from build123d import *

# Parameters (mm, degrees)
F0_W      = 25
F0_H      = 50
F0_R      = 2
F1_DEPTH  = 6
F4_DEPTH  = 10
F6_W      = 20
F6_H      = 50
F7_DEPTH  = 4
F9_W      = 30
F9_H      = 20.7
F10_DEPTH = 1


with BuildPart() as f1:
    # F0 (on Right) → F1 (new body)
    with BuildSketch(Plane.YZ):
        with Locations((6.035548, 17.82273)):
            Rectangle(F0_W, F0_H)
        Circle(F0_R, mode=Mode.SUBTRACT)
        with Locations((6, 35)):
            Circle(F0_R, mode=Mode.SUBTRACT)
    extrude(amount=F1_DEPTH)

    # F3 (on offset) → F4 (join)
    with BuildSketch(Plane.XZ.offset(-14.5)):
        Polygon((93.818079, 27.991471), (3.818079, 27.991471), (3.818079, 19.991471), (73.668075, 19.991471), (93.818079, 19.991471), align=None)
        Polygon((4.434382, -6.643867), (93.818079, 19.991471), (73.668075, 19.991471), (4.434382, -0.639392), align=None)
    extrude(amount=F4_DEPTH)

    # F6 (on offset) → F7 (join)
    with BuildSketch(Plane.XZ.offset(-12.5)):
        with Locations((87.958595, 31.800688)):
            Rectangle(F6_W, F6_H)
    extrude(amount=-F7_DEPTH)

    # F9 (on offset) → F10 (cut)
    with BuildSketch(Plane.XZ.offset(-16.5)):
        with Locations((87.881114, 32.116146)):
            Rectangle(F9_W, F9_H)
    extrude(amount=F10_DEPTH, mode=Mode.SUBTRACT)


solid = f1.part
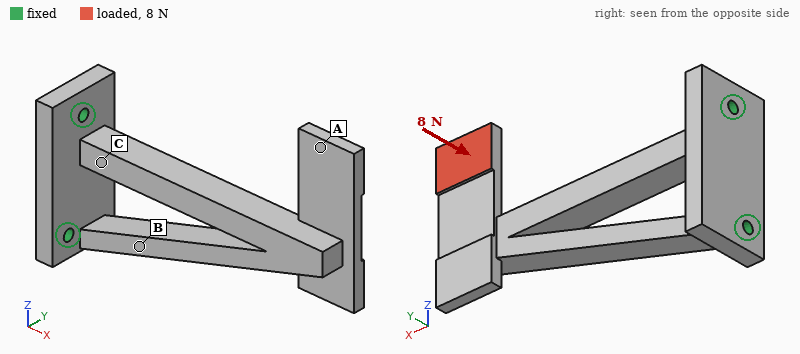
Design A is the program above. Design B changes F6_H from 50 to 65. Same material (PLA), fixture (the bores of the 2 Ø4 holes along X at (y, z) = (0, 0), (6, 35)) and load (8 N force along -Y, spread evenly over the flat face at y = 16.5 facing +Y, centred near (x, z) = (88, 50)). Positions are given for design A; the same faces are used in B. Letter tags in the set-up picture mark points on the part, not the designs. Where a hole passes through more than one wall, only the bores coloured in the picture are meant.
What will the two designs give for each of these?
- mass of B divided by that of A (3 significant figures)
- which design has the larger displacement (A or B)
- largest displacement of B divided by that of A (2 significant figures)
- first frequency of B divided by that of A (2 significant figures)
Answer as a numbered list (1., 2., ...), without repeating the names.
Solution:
1. 1.05
2. B
3. 1.2
4. 0.91
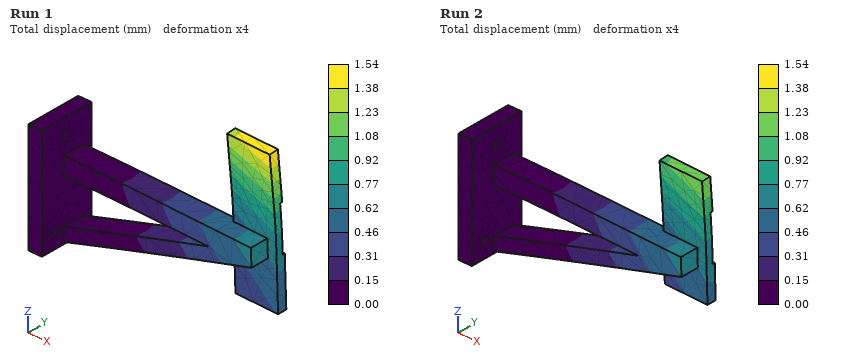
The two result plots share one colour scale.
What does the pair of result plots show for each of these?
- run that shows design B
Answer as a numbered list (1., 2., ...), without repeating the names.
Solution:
1. Run 1
